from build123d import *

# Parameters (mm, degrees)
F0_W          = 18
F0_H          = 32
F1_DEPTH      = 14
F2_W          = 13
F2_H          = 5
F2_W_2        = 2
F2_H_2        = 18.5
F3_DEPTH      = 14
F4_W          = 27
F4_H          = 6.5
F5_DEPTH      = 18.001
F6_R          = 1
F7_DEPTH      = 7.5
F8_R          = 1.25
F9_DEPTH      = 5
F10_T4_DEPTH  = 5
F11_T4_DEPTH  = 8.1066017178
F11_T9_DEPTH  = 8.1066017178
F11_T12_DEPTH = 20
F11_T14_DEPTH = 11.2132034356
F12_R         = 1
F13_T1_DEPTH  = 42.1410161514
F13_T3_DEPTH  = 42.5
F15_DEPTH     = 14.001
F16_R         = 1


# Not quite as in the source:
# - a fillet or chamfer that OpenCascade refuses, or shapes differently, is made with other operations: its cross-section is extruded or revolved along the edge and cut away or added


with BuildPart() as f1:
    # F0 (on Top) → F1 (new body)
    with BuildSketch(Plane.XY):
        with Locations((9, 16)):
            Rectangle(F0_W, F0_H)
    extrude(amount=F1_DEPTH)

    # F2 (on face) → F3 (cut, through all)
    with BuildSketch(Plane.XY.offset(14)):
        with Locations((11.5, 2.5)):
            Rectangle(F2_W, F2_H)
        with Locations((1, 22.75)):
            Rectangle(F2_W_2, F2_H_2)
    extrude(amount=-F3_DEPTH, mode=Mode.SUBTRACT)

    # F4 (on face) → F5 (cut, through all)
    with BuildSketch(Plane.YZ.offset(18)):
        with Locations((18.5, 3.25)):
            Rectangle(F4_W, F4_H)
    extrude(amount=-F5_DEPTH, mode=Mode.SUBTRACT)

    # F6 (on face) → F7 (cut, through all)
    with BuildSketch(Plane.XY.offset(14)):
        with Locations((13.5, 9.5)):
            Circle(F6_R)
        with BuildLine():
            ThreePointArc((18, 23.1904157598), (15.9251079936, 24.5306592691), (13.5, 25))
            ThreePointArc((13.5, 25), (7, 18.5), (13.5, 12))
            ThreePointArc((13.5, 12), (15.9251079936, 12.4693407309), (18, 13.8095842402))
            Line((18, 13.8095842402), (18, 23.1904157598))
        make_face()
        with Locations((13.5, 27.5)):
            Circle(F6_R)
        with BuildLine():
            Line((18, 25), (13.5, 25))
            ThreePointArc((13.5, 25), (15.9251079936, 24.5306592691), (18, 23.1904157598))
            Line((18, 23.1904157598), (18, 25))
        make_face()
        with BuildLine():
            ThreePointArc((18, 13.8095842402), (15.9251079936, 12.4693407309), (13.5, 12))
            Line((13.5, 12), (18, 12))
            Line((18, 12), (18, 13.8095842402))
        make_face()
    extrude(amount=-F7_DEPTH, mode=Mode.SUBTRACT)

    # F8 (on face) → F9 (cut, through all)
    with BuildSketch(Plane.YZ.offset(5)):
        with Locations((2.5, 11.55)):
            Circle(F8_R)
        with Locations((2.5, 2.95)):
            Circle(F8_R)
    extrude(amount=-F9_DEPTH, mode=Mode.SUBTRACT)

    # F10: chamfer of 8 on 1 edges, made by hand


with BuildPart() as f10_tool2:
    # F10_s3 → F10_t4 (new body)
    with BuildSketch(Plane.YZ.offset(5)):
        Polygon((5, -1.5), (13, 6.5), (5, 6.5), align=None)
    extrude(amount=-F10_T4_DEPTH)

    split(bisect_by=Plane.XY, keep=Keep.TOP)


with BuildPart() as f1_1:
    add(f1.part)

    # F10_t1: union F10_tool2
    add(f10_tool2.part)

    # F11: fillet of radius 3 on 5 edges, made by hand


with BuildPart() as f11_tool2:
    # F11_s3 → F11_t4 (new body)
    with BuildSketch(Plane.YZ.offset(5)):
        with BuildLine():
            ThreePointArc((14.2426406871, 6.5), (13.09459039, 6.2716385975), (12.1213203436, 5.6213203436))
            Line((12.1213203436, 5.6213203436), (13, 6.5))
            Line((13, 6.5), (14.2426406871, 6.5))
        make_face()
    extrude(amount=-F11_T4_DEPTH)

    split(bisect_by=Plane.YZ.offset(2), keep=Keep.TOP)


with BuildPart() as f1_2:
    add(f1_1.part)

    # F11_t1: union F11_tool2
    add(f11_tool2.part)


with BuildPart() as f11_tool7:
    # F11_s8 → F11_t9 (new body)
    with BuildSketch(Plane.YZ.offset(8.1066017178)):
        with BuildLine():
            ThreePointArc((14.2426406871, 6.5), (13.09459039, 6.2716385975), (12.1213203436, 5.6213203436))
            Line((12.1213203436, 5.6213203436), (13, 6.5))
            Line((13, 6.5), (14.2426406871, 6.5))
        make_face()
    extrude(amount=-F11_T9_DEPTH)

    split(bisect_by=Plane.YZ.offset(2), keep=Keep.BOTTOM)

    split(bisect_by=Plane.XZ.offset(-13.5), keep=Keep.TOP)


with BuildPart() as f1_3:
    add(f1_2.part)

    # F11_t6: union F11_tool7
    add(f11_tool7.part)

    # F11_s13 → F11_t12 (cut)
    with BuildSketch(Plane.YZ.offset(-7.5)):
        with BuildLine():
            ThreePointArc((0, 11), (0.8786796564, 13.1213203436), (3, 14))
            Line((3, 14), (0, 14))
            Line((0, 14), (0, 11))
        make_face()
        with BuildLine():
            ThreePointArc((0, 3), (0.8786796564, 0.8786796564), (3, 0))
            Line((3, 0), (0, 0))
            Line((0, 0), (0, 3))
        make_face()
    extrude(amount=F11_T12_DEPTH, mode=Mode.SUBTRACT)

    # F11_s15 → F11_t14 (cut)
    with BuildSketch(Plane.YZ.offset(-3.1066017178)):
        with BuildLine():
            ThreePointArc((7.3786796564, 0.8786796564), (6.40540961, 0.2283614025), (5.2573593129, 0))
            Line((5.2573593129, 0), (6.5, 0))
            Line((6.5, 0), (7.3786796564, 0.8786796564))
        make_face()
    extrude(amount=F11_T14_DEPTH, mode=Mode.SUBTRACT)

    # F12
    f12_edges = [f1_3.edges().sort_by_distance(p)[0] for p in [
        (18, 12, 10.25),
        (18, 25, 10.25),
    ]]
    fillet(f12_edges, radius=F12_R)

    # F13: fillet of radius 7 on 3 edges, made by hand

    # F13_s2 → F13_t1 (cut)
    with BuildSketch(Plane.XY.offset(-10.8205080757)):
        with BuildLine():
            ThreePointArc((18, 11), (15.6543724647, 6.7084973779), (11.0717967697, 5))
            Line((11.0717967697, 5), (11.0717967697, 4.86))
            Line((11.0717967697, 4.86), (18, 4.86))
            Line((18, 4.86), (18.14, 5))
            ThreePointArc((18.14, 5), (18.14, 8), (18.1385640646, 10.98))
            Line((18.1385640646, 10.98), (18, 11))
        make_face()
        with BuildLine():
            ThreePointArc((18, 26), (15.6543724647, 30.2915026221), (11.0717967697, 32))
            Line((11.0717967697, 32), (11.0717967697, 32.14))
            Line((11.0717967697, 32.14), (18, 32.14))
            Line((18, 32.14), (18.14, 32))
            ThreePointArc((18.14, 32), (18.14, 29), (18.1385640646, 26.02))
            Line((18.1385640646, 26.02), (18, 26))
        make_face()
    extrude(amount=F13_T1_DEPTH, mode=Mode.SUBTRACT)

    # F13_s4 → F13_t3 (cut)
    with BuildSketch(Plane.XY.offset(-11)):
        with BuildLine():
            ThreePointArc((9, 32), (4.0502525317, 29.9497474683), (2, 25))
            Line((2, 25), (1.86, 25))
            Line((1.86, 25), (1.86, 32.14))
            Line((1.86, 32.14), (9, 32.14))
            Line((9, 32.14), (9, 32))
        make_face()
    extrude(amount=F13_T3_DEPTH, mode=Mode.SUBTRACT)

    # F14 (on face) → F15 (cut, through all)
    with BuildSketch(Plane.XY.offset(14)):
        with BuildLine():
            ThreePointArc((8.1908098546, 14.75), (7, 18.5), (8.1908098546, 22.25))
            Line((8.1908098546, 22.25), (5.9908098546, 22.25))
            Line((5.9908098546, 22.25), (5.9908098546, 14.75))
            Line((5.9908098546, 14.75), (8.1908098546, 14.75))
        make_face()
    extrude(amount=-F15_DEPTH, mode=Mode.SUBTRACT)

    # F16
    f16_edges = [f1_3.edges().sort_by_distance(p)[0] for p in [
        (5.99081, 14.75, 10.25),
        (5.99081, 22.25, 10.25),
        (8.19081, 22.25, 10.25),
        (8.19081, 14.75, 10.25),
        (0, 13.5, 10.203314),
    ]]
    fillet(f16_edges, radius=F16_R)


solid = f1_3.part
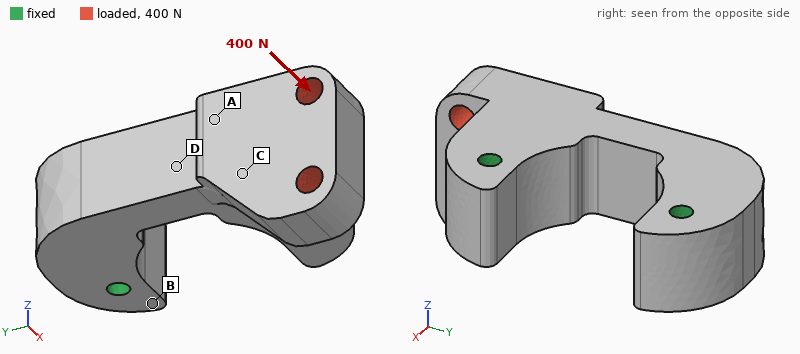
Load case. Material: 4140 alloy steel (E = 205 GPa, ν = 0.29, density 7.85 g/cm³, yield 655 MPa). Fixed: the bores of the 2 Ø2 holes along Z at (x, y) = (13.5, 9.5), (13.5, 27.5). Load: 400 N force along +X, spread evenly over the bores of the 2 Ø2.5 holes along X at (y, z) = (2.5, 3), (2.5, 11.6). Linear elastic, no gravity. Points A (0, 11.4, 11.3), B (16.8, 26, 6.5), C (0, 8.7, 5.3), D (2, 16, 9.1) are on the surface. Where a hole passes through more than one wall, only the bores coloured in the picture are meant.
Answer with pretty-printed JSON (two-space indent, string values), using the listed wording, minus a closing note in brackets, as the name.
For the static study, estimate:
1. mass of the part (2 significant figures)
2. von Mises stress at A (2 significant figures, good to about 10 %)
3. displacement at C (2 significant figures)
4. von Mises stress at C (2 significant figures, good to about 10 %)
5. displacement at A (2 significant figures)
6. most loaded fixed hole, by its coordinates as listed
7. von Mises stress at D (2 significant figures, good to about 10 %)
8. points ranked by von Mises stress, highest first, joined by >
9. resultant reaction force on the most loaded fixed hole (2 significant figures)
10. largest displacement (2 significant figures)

{
  "mass of the part": "20 g",
  "von Mises stress at A": "8.3 MPa",
  "displacement at C": "3.1 µm",
  "von Mises stress at C": "24 MPa",
  "displacement at A": "2.3 µm",
  "most loaded fixed hole, by its coordinates as listed": "(13.5, 9.5)",
  "von Mises stress at D": "20 MPa",
  "points ranked by von Mises stress, highest first, joined by >": "C > D > A > B",
  "resultant reaction force on the most loaded fixed hole": "520 N",
  "largest displacement": "7.5 µm"
}
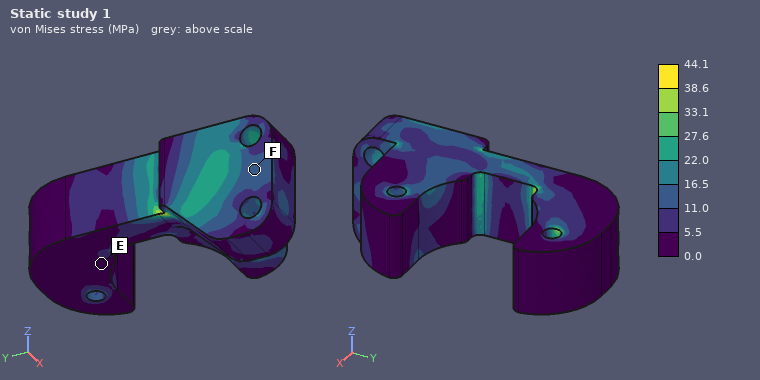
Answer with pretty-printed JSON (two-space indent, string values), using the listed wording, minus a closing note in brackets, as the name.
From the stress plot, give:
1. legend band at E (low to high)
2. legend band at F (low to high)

{
  "legend band at E": "0.0 to 5.5 MPa",
  "legend band at F": "11.0 to 16.5 MPa"
}
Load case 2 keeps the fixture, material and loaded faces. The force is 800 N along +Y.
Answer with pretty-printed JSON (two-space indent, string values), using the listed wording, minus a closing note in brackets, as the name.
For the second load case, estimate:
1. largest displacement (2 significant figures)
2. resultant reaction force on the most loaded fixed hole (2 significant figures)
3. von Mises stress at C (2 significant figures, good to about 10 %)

{
  "largest displacement": "9.8 µm",
  "resultant reaction force on the most loaded fixed hole": "530 N",
  "von Mises stress at C": "19 MPa"
}
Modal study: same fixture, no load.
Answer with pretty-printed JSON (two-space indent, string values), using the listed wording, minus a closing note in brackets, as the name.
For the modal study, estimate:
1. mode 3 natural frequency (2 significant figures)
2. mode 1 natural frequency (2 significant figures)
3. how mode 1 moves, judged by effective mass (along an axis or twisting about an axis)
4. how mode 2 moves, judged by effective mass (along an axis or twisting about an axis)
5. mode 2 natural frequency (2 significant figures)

{
  "mode 3 natural frequency": "28 kHz",
  "mode 1 natural frequency": "16 kHz",
  "how mode 1 moves, judged by effective mass": "along Z",
  "how mode 2 moves, judged by effective mass": "along Y",
  "mode 2 natural frequency": "20 kHz"
}
